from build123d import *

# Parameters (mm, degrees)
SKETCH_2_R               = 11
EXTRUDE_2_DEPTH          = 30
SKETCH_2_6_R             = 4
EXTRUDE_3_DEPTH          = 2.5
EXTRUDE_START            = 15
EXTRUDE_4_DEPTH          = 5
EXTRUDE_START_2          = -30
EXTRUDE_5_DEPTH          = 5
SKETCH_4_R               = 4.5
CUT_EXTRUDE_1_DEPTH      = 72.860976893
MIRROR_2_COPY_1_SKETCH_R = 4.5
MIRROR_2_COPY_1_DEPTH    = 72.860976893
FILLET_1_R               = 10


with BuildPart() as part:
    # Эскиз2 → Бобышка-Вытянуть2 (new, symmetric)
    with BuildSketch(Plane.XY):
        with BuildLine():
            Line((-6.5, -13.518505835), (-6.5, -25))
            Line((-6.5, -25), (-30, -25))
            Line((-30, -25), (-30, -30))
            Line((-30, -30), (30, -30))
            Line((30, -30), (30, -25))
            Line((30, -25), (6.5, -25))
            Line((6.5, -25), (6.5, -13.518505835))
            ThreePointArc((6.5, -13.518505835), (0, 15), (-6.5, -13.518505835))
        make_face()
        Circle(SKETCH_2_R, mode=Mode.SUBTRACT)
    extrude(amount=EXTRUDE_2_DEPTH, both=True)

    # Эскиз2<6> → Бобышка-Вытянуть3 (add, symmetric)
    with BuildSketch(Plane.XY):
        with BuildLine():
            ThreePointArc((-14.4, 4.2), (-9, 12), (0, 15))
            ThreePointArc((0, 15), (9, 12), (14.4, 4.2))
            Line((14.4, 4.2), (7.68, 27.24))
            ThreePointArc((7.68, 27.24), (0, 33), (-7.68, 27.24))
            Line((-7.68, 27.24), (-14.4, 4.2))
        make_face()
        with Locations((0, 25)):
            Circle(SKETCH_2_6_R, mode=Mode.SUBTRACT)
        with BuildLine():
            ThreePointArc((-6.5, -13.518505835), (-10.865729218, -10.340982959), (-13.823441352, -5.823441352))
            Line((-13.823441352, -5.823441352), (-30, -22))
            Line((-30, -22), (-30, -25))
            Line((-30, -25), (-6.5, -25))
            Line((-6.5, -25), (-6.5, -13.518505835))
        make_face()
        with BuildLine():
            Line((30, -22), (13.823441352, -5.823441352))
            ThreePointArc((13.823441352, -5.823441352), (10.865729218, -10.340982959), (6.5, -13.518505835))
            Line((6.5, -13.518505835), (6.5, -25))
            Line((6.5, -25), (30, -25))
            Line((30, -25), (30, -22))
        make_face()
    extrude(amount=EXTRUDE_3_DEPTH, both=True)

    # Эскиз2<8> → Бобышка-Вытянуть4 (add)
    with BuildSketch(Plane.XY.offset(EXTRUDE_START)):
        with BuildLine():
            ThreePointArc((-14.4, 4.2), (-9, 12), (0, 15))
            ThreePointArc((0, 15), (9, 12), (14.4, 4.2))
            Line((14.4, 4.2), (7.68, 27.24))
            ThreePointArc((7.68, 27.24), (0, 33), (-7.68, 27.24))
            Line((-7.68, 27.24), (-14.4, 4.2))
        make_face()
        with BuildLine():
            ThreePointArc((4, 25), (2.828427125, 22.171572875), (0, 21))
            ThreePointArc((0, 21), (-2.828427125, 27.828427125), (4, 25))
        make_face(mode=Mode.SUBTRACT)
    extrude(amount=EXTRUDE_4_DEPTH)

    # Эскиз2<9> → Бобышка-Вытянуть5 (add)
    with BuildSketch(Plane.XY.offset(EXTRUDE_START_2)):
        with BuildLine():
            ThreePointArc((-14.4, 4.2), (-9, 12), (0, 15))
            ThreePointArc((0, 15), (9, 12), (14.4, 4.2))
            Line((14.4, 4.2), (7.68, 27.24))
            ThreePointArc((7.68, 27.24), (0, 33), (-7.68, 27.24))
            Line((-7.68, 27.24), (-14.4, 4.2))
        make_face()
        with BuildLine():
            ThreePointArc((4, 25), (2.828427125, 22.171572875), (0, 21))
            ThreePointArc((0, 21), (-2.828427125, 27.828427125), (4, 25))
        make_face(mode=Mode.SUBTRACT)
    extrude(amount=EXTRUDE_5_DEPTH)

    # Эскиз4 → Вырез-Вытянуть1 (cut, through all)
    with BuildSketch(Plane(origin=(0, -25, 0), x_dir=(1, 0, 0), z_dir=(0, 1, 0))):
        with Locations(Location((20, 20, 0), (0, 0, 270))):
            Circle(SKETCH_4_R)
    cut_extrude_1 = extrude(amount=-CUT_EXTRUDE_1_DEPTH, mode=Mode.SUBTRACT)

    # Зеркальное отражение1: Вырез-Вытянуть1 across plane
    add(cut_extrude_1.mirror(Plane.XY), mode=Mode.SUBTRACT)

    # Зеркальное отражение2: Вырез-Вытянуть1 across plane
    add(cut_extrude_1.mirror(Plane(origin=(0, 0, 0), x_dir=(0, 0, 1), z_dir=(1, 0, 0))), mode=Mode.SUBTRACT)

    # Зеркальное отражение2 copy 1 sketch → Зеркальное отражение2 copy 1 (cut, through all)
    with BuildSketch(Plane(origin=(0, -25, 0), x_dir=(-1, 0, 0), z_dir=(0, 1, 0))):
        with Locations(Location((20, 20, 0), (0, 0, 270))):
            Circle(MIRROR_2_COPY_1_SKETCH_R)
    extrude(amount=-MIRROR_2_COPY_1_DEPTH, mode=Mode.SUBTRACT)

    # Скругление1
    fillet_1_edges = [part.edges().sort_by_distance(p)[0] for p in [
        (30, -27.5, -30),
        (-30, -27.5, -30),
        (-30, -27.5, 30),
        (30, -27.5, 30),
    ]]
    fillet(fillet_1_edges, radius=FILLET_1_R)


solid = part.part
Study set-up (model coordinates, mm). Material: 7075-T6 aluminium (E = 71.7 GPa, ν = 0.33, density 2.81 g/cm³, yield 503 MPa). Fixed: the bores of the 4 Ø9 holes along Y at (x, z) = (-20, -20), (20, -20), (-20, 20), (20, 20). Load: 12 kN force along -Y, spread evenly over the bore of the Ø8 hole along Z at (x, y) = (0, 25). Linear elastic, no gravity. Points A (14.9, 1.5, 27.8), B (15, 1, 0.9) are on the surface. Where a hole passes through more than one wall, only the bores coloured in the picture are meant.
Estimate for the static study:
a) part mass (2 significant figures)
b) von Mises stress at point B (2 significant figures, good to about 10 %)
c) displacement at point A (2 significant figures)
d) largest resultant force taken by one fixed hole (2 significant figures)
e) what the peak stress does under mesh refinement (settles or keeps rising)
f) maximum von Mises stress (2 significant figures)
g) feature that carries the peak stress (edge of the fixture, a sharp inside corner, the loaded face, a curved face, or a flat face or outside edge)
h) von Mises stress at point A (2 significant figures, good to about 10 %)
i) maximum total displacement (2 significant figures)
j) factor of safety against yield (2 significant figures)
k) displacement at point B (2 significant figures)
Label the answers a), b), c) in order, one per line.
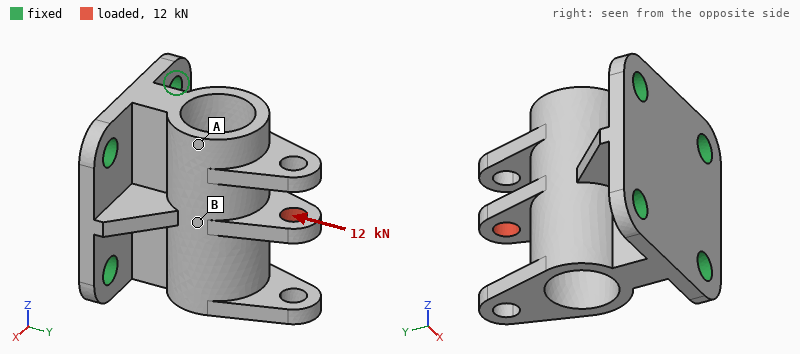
a) 140 g
b) 58 MPa
c) 0.049 mm
d) 3.1 kN
e) settles
f) 320 MPa
g) the loaded face
h) 30 MPa
i) 0.14 mm
j) 1.6
k) 0.067 mm
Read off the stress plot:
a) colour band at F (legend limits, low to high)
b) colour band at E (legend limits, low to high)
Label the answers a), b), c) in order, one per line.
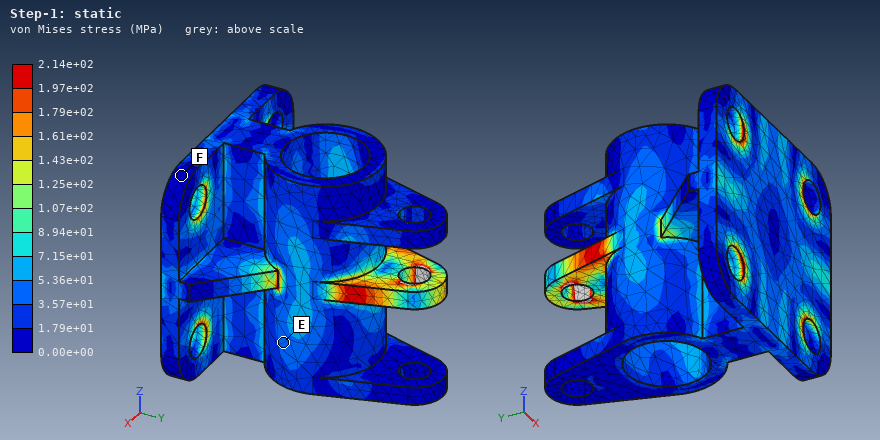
a) 0.00e+00 to 1.79e+01 MPa
b) 3.57e+01 to 5.36e+01 MPa
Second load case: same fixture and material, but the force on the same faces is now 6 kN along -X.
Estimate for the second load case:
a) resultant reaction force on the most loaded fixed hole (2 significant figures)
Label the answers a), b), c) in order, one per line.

a) 4.7 kN
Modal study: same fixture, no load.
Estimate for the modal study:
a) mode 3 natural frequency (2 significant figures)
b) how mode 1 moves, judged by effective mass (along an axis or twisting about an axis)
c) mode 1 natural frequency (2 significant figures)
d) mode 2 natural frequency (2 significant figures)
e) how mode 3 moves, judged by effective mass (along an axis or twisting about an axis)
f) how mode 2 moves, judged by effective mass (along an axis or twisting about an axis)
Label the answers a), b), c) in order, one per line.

a) 7800 Hz
b) along X
c) 3500 Hz
d) 4200 Hz
e) along Y
f) along Z
